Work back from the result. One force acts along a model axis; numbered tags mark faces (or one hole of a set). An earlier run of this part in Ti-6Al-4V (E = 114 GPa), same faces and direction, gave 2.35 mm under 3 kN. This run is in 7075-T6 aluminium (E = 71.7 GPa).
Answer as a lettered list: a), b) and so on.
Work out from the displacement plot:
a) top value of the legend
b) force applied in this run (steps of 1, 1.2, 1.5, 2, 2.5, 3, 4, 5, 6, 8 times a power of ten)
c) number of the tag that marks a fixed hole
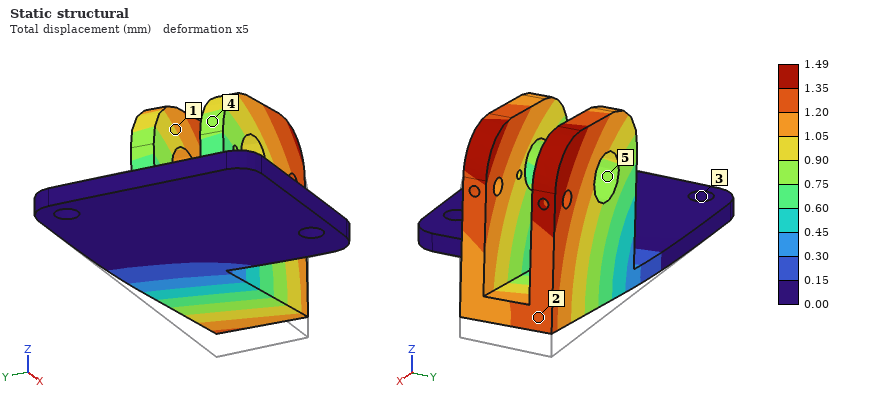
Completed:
a) 1.49 mm
b) 1.2 kN
c) 3
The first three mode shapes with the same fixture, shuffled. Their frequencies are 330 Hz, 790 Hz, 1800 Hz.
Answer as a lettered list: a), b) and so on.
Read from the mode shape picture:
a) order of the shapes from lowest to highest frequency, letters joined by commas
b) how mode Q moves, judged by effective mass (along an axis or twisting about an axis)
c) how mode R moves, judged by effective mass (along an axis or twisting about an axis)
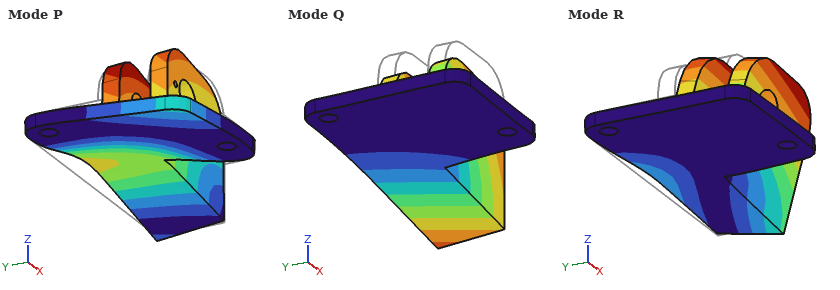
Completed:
a) Q, R, P
b) along Z
c) along Y
